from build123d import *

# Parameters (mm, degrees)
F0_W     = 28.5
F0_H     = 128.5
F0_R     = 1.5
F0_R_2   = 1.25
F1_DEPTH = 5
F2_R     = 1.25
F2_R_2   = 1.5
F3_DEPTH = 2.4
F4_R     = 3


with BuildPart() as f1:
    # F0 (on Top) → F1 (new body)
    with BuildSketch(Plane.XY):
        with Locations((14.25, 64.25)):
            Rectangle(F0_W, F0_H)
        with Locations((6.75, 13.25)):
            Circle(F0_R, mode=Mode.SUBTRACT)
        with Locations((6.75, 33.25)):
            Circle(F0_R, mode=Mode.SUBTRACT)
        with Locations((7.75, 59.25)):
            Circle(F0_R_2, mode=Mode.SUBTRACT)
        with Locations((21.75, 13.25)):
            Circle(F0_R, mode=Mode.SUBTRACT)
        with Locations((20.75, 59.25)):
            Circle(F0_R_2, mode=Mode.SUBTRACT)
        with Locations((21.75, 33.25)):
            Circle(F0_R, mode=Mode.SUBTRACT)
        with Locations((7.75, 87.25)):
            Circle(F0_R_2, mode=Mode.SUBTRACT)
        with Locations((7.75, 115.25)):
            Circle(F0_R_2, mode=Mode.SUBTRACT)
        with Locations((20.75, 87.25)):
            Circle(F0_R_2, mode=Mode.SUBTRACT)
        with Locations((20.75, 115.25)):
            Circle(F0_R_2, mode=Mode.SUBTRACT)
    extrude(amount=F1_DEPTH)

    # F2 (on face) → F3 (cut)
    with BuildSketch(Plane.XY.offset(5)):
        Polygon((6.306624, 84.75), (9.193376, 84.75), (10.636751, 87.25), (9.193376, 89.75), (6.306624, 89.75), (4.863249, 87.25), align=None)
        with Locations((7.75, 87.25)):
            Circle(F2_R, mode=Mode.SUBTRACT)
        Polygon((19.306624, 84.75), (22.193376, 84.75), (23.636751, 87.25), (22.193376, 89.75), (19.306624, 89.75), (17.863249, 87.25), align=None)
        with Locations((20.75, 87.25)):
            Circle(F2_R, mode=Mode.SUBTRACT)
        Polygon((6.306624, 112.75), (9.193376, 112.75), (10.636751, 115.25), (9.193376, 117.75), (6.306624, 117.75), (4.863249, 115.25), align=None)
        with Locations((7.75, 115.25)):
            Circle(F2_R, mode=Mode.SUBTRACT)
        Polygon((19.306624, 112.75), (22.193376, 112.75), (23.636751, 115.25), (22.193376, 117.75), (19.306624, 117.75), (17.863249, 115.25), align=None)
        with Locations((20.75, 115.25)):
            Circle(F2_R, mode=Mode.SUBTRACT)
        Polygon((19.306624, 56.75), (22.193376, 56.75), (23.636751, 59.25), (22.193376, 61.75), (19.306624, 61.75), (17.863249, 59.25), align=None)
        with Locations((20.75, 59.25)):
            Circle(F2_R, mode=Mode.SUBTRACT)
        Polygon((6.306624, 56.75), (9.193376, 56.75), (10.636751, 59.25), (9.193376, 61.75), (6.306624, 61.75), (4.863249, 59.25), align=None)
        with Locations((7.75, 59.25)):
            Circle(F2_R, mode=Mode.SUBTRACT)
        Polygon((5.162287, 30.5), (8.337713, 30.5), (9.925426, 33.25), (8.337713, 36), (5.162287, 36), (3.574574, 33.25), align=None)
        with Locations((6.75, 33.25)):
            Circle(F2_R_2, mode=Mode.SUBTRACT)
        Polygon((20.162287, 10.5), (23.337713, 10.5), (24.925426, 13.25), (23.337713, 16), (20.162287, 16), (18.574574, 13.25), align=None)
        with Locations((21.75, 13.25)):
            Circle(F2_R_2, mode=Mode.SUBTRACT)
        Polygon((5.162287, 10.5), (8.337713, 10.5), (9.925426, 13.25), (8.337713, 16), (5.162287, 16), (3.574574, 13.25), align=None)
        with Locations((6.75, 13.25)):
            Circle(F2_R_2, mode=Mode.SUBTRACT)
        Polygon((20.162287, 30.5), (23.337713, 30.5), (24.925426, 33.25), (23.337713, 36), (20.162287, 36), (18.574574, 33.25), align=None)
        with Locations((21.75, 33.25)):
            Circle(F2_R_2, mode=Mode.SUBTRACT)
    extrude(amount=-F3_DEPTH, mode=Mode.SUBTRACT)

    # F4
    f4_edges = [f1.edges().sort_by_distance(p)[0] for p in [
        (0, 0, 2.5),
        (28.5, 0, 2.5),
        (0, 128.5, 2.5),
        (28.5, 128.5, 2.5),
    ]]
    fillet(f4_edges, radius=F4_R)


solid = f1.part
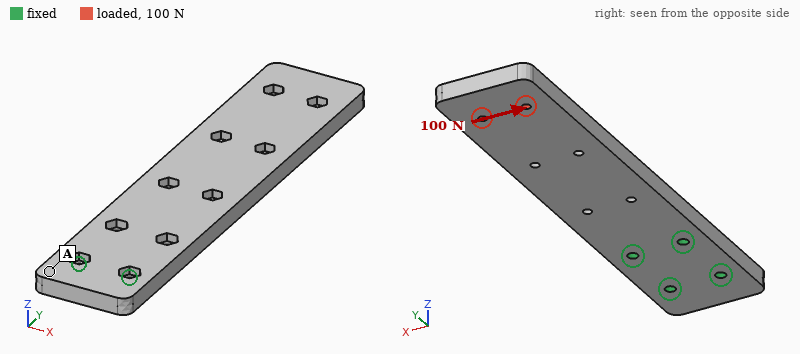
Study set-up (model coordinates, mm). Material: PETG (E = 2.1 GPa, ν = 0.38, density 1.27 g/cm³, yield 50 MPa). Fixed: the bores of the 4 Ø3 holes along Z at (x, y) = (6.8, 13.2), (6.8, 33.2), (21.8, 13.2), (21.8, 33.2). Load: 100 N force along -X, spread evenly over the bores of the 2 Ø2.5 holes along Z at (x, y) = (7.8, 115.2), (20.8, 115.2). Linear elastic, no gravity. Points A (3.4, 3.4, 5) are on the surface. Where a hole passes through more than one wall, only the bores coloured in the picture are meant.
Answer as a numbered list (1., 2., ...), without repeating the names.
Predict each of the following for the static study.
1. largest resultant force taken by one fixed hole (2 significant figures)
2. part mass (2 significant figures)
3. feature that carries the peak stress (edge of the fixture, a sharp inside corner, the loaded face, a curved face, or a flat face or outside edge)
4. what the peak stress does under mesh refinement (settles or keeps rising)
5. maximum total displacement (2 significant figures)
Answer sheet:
1. 340 N
2. 22 g
3. edge of the fixture
4. keeps rising
5. 1.6 mm
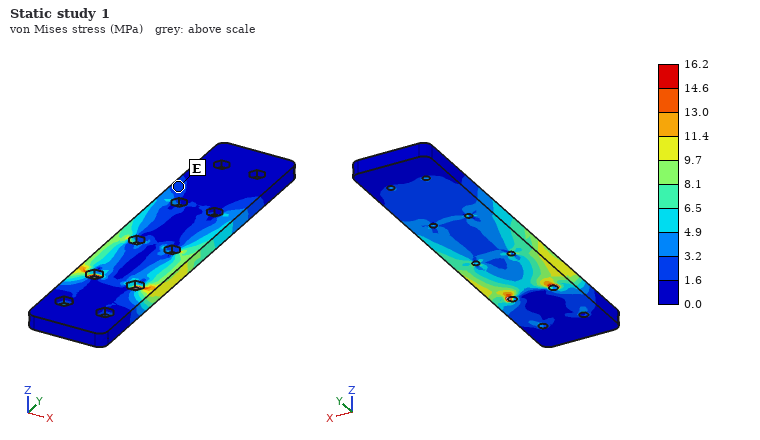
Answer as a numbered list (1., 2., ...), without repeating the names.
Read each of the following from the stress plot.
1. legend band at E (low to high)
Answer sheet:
1. 1.6 to 3.2 MPa
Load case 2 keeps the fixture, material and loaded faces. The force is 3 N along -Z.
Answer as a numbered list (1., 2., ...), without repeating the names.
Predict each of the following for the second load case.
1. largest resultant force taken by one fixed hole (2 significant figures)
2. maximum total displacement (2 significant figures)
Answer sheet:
1. 11 N
2. 1.3 mm
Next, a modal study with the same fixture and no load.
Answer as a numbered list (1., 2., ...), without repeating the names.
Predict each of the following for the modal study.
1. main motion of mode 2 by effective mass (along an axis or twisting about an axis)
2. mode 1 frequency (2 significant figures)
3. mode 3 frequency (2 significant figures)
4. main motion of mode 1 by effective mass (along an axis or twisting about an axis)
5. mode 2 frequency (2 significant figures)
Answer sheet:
1. along X
2. 110 Hz
3. 660 Hz
4. along Z
5. 550 Hz
